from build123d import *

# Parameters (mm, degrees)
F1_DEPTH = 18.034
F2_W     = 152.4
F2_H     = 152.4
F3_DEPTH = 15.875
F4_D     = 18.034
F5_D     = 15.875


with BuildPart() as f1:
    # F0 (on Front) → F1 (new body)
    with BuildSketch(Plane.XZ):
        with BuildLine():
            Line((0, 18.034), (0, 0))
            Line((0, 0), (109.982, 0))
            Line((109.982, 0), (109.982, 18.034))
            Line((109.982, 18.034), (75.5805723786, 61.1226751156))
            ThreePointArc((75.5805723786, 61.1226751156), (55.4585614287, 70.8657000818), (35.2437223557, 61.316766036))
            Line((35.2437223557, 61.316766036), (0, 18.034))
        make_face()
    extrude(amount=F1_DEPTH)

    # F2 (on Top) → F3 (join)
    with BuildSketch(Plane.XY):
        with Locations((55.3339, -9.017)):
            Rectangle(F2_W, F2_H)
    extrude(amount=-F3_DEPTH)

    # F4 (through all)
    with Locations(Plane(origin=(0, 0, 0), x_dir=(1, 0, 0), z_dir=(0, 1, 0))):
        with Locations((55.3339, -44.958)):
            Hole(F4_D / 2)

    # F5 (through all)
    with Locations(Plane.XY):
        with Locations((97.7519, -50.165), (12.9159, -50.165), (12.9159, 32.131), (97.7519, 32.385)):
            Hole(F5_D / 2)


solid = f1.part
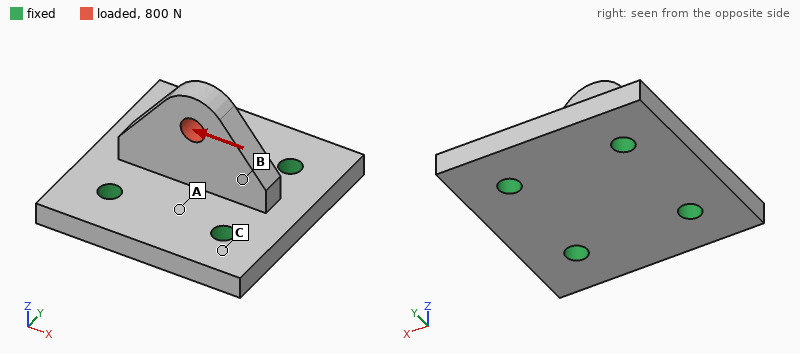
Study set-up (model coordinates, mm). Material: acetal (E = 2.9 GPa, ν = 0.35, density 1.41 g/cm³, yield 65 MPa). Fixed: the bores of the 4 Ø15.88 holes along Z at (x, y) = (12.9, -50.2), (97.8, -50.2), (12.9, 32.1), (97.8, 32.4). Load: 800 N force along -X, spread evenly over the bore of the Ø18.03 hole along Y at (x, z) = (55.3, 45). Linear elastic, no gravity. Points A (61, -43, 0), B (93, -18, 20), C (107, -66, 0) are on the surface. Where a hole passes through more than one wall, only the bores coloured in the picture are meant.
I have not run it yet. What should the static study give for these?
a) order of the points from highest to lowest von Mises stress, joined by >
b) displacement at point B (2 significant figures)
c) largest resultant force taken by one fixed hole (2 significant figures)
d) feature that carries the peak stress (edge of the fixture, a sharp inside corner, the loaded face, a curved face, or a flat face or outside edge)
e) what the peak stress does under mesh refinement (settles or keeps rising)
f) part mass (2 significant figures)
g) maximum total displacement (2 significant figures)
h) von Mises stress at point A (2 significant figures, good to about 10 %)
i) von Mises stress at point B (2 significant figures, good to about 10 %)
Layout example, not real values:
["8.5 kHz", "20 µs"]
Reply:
["B > A > C", "37 µm", "310 N", "edge of the fixture", "keeps rising", "640 g", "78 µm", "0.51 MPa", "0.83 MPa"]
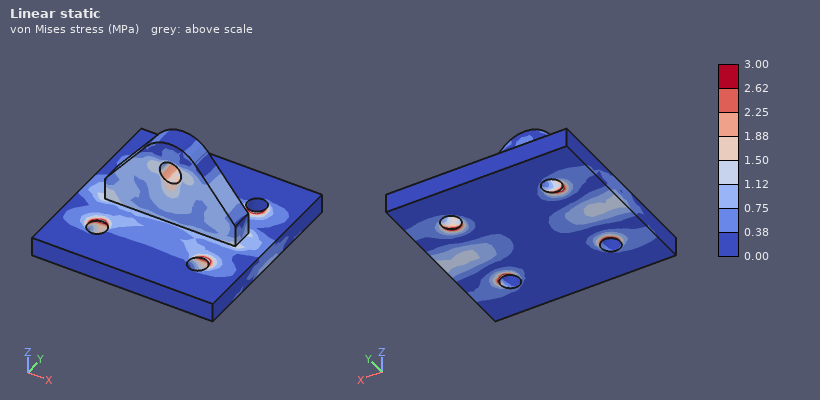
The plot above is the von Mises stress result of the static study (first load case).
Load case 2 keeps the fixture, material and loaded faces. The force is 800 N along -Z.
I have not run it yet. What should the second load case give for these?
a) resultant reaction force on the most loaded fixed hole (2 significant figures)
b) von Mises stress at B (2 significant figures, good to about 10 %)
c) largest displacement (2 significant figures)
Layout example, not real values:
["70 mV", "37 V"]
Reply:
["210 N", "0.48 MPa", "39 µm"]
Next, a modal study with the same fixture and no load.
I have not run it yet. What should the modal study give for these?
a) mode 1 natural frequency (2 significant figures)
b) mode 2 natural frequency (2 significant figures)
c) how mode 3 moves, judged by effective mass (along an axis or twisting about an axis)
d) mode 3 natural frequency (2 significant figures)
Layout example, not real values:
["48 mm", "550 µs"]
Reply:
["950 Hz", "1800 Hz", "along Z", "1900 Hz"]
